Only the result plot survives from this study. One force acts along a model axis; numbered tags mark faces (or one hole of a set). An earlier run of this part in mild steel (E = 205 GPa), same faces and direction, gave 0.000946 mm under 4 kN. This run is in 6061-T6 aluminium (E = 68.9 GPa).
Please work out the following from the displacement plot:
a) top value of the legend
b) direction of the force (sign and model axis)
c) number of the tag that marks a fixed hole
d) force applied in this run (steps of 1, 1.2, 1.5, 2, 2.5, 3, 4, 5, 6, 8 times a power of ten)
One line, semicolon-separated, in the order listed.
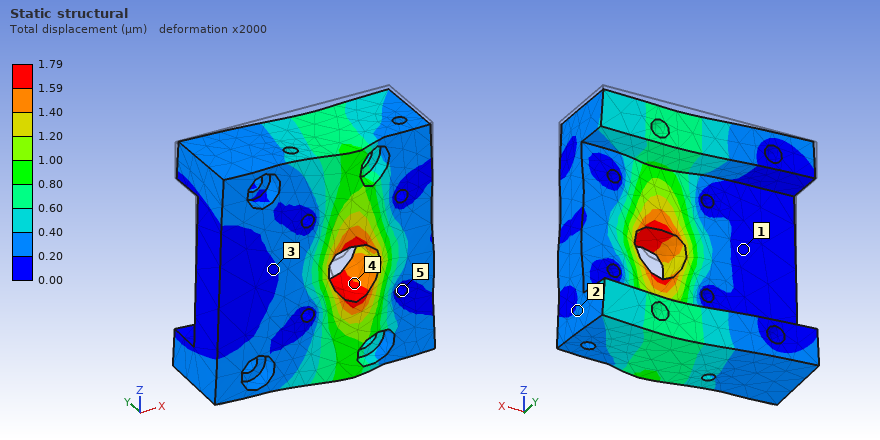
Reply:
1.79 µm; -Z; 5; 2.5 kN
